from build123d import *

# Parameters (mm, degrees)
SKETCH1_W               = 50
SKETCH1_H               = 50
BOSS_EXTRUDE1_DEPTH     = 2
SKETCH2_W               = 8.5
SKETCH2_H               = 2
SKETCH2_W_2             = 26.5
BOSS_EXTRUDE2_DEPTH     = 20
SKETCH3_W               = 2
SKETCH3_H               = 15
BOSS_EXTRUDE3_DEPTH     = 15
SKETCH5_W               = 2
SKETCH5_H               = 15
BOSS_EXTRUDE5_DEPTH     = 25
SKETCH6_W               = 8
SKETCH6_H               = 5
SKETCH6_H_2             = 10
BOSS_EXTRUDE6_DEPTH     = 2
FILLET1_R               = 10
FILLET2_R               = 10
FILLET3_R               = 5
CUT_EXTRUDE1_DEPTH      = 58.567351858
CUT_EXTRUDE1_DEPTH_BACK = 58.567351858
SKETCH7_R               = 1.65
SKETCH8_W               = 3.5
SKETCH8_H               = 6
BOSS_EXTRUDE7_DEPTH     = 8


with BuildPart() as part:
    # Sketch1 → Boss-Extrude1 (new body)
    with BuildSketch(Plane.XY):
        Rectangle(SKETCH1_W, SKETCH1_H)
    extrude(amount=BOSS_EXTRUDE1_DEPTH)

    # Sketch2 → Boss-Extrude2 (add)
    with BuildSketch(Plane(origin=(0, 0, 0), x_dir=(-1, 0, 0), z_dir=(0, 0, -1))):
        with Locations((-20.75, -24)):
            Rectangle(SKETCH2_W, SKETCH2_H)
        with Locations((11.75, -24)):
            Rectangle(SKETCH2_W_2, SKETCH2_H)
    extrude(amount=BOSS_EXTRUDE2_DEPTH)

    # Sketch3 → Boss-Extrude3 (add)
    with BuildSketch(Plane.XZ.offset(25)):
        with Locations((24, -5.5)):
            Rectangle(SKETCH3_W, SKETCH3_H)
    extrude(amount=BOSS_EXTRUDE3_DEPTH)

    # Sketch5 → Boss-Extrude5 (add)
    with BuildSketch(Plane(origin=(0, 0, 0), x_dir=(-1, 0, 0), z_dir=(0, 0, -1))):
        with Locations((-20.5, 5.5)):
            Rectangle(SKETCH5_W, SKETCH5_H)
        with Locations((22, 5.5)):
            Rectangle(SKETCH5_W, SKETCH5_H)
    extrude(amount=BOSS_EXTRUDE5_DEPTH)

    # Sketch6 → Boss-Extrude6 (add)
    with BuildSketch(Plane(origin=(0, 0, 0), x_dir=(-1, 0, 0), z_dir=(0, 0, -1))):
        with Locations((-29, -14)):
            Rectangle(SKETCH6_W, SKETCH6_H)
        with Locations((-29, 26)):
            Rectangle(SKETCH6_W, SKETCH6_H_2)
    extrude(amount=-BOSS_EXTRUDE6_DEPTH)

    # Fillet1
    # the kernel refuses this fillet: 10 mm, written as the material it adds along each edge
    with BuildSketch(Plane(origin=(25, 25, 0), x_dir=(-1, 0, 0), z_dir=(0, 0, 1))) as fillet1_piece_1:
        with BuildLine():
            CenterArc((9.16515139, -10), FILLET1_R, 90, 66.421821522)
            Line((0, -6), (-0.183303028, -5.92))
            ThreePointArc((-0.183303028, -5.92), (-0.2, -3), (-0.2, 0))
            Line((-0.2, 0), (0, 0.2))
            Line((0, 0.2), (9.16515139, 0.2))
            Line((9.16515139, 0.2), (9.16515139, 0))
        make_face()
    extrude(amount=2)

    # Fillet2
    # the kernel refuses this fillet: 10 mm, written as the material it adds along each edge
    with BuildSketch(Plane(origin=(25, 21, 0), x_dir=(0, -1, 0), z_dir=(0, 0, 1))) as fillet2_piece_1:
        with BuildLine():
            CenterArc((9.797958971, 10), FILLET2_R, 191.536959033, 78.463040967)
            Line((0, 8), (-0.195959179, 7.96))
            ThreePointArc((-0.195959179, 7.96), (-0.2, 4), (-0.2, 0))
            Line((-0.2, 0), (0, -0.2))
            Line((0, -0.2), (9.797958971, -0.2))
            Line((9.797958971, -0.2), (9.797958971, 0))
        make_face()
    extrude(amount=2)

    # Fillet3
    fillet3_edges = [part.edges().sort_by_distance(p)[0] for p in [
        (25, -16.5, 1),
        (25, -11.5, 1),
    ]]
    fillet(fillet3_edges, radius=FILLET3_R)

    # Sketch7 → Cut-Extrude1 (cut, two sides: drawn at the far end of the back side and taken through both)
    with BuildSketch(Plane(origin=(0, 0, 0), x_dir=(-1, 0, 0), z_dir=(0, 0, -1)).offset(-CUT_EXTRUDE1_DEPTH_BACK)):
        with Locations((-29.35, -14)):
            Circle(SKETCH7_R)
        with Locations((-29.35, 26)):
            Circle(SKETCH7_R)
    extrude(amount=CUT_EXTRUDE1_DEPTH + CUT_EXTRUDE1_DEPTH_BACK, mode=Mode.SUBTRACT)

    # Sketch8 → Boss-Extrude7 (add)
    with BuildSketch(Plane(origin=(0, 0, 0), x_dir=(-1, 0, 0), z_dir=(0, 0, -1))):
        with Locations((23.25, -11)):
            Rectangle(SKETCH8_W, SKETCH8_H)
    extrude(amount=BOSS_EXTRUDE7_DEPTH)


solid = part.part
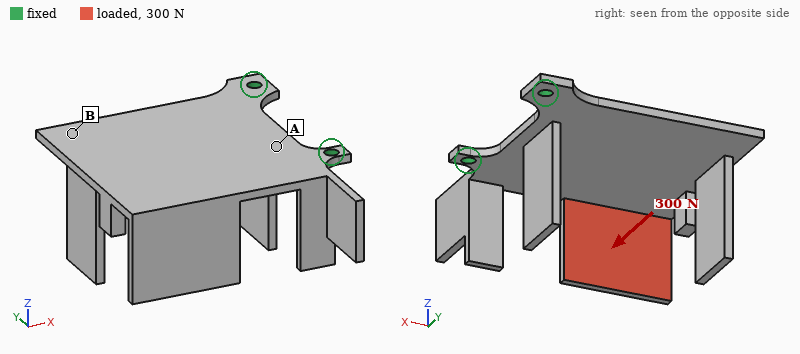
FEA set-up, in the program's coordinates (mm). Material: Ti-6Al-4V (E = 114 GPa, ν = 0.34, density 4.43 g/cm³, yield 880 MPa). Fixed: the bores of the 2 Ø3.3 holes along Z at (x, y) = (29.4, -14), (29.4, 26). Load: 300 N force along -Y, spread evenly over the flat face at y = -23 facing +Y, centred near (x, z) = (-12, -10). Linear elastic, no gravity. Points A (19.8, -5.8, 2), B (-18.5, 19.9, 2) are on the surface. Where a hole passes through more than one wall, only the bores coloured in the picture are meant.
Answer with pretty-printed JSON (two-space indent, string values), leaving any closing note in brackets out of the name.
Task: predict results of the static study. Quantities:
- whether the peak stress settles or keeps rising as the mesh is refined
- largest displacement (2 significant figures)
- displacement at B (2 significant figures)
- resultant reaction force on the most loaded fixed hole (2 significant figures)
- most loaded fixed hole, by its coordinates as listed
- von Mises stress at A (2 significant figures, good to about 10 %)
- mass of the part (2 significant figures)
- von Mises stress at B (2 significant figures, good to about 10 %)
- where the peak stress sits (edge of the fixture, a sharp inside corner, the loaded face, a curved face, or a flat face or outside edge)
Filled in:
{
  "whether the peak stress settles or keeps rising as the mesh is refined": "keeps rising",
  "largest displacement": "0.98 mm",
  "displacement at B": "0.30 mm",
  "resultant reaction force on the most loaded fixed hole": "380 N",
  "most loaded fixed hole, by its coordinates as listed": "(29.4, 26)",
  "von Mises stress at A": "61 MPa",
  "mass of the part": "39 g",
  "von Mises stress at B": "25 MPa",
  "where the peak stress sits": "edge of the fixture"
}
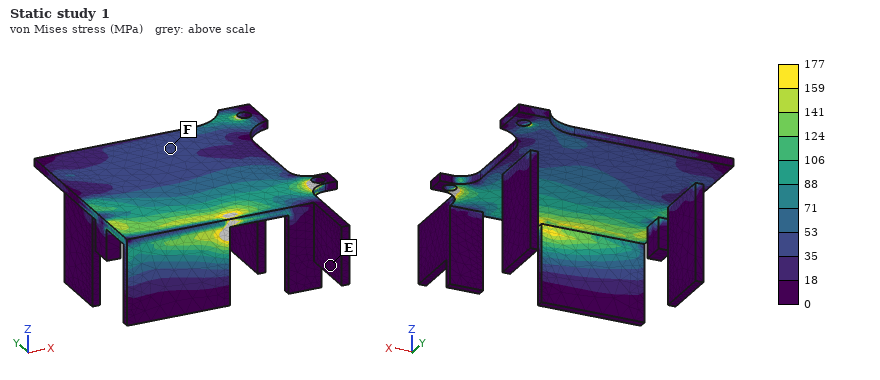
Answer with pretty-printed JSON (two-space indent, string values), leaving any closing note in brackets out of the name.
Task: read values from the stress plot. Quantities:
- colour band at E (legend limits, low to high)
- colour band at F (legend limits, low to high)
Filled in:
{
  "colour band at E": "0 to 18 MPa",
  "colour band at F": "35 to 53 MPa"
}
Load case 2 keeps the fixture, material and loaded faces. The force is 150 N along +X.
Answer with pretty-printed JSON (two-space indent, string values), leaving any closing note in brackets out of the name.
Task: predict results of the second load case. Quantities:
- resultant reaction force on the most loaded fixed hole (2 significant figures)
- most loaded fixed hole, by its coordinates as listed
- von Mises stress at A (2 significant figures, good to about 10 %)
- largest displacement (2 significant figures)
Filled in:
{
  "resultant reaction force on the most loaded fixed hole": "180 N",
  "most loaded fixed hole, by its coordinates as listed": "(29.4, -14)",
  "von Mises stress at A": "38 MPa",
  "largest displacement": "1.1 mm"
}
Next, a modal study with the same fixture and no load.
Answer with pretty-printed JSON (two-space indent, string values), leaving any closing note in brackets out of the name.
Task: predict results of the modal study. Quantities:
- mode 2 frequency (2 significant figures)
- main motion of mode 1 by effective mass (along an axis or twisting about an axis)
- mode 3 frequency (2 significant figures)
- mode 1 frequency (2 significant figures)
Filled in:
{
  "mode 2 frequency": "850 Hz",
  "main motion of mode 1 by effective mass": "along Z",
  "mode 3 frequency": "1500 Hz",
  "mode 1 frequency": "290 Hz"
}
